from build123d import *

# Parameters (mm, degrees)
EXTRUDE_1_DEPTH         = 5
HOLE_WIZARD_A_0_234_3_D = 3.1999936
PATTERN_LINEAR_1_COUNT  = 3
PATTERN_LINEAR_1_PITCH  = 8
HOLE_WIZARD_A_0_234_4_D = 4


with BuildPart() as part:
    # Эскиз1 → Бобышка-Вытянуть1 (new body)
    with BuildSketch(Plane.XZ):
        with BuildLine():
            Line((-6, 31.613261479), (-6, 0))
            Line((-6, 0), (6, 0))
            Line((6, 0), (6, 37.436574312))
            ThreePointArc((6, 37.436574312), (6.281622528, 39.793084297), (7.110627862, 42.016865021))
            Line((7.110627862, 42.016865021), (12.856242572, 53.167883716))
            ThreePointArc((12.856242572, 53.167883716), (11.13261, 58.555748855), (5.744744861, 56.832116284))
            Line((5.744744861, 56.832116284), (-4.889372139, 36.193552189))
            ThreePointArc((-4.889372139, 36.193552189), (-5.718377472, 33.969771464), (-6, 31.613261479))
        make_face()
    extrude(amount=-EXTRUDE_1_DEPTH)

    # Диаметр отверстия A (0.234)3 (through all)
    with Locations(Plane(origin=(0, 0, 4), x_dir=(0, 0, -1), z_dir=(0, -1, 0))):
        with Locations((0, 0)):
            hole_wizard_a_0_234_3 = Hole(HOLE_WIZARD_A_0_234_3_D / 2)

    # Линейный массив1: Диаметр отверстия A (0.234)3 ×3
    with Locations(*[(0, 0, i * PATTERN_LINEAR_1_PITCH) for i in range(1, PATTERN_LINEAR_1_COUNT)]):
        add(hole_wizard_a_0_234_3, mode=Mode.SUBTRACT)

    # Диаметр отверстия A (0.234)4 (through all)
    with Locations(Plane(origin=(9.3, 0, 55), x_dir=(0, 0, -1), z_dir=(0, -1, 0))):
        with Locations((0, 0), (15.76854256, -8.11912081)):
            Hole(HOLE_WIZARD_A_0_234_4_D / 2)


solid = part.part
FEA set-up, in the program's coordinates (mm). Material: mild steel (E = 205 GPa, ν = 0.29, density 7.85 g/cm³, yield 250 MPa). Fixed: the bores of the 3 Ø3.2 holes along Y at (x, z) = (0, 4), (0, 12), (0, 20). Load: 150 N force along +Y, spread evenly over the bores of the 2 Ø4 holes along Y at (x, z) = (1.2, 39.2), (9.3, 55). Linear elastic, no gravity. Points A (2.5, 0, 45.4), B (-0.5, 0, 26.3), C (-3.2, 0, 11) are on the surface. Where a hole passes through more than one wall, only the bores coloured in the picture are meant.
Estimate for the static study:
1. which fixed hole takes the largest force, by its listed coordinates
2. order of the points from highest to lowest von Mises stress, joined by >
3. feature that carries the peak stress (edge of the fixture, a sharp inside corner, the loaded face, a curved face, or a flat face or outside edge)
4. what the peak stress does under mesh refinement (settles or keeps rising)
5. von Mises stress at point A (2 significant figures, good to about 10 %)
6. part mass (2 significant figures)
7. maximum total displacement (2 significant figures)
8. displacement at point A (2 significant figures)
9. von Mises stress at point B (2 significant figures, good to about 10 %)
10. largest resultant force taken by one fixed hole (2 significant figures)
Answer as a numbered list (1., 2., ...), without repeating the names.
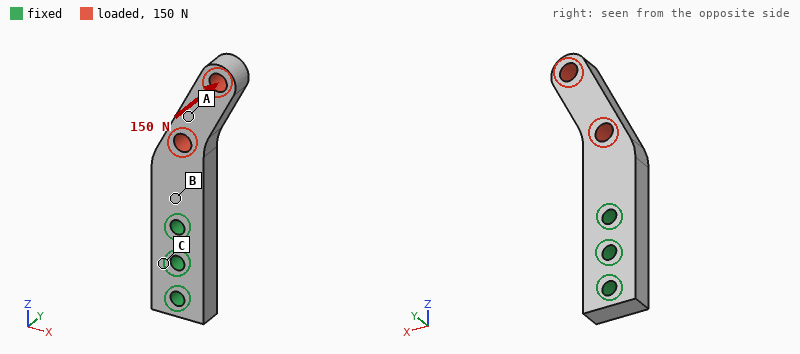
1. (0, 20)
2. B > A > C
3. edge of the fixture
4. keeps rising
5. 24 MPa
6. 23 g
7. 85 µm
8. 40 µm
9. 64 MPa
10. 270 N
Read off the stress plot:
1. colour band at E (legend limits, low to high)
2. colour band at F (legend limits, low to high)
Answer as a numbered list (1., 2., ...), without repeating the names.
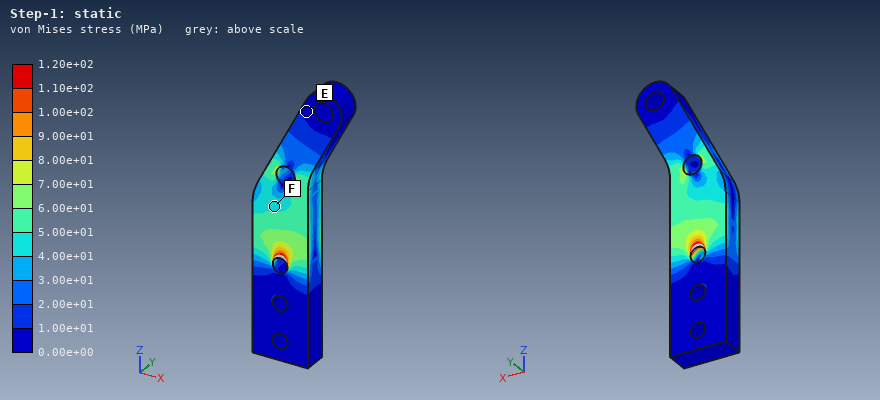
1. 0.00e+00 to 1.00e+01 MPa
2. 4.00e+01 to 5.00e+01 MPa
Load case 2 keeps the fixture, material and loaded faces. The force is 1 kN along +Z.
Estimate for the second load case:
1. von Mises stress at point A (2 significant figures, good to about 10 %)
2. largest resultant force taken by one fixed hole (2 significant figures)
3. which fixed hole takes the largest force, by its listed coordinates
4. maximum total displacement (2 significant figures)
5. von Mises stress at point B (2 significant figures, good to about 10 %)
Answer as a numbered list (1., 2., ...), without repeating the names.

1. 14 MPa
2. 880 N
3. (0, 20)
4. 42 µm
5. 16 MPa
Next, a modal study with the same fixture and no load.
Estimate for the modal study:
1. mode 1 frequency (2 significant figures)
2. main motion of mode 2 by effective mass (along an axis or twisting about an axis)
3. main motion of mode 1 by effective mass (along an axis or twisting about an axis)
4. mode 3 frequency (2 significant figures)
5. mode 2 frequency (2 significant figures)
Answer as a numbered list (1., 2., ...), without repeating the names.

1. 3200 Hz
2. along X
3. along Y
4. 14 kHz
5. 6200 Hz
